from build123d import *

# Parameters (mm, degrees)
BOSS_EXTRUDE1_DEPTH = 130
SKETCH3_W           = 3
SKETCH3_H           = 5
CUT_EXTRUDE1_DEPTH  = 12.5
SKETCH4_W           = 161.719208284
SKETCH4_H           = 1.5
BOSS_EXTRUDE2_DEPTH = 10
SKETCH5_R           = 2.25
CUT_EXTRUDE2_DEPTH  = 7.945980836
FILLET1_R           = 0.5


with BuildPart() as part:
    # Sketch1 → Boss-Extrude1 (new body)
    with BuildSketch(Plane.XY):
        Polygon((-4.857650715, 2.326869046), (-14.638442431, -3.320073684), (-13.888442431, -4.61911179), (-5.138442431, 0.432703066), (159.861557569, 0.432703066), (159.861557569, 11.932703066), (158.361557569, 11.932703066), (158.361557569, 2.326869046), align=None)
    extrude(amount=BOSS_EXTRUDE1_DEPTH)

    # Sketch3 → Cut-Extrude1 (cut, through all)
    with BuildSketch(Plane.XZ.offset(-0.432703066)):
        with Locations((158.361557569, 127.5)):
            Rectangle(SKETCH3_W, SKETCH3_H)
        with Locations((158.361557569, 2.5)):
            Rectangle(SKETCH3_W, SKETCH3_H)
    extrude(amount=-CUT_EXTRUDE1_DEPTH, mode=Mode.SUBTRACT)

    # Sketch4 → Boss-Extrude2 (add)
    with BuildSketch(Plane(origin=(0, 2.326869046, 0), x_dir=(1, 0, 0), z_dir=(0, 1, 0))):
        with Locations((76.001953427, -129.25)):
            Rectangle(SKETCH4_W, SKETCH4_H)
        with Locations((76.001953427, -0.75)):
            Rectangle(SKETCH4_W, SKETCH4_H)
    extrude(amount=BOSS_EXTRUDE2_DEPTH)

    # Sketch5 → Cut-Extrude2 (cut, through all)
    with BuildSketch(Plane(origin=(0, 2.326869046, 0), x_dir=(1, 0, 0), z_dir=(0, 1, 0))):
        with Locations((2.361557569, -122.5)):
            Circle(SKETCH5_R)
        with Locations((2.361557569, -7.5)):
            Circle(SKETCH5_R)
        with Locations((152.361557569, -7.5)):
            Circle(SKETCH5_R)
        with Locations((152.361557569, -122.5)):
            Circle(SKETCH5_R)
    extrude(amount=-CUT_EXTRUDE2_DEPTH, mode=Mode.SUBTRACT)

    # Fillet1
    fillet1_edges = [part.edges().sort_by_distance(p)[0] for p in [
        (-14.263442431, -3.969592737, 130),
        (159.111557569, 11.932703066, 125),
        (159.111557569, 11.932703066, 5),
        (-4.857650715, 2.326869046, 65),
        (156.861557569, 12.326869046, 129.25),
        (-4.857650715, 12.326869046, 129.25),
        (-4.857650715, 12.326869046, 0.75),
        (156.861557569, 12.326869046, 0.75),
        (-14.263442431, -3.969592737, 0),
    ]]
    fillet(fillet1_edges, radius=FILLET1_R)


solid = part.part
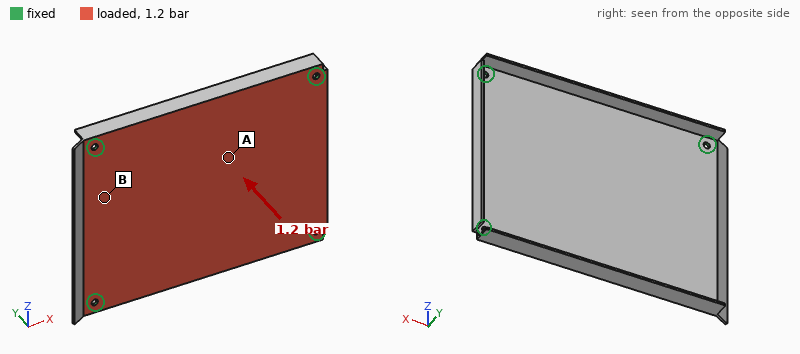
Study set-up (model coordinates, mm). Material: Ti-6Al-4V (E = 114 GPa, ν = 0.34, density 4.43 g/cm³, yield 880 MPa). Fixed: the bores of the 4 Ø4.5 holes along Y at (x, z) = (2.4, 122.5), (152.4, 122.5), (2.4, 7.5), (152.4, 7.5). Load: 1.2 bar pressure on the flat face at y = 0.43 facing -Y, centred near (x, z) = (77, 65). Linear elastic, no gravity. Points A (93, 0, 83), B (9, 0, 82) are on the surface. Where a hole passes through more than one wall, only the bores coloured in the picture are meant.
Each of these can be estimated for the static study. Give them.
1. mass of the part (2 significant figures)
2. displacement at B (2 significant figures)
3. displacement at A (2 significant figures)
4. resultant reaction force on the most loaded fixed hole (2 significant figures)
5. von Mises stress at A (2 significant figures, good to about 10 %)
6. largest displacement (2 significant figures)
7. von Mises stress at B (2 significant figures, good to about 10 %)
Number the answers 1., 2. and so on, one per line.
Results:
1. 220 g
2. 0.76 mm
3. 2.2 mm
4. 1.1 kN
5. 160 MPa
6. 2.5 mm
7. 77 MPa
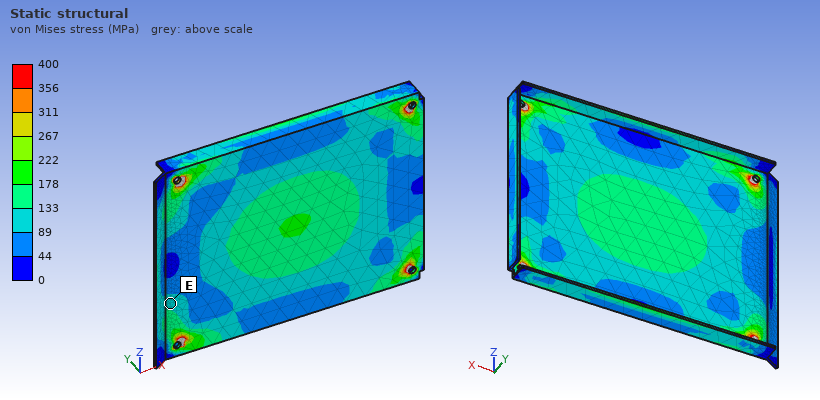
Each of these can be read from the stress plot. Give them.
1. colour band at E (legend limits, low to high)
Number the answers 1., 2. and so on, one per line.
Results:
1. 89 to 133 MPa
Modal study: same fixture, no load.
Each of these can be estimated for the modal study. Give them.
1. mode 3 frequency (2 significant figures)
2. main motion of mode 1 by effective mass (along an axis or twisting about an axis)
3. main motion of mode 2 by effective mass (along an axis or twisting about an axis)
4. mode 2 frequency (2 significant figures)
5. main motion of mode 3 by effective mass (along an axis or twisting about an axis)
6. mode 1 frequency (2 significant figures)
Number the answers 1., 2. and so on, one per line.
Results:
1. 1100 Hz
2. along Y
3. twisting about Z
4. 990 Hz
5. twisting about X
6. 480 Hz
